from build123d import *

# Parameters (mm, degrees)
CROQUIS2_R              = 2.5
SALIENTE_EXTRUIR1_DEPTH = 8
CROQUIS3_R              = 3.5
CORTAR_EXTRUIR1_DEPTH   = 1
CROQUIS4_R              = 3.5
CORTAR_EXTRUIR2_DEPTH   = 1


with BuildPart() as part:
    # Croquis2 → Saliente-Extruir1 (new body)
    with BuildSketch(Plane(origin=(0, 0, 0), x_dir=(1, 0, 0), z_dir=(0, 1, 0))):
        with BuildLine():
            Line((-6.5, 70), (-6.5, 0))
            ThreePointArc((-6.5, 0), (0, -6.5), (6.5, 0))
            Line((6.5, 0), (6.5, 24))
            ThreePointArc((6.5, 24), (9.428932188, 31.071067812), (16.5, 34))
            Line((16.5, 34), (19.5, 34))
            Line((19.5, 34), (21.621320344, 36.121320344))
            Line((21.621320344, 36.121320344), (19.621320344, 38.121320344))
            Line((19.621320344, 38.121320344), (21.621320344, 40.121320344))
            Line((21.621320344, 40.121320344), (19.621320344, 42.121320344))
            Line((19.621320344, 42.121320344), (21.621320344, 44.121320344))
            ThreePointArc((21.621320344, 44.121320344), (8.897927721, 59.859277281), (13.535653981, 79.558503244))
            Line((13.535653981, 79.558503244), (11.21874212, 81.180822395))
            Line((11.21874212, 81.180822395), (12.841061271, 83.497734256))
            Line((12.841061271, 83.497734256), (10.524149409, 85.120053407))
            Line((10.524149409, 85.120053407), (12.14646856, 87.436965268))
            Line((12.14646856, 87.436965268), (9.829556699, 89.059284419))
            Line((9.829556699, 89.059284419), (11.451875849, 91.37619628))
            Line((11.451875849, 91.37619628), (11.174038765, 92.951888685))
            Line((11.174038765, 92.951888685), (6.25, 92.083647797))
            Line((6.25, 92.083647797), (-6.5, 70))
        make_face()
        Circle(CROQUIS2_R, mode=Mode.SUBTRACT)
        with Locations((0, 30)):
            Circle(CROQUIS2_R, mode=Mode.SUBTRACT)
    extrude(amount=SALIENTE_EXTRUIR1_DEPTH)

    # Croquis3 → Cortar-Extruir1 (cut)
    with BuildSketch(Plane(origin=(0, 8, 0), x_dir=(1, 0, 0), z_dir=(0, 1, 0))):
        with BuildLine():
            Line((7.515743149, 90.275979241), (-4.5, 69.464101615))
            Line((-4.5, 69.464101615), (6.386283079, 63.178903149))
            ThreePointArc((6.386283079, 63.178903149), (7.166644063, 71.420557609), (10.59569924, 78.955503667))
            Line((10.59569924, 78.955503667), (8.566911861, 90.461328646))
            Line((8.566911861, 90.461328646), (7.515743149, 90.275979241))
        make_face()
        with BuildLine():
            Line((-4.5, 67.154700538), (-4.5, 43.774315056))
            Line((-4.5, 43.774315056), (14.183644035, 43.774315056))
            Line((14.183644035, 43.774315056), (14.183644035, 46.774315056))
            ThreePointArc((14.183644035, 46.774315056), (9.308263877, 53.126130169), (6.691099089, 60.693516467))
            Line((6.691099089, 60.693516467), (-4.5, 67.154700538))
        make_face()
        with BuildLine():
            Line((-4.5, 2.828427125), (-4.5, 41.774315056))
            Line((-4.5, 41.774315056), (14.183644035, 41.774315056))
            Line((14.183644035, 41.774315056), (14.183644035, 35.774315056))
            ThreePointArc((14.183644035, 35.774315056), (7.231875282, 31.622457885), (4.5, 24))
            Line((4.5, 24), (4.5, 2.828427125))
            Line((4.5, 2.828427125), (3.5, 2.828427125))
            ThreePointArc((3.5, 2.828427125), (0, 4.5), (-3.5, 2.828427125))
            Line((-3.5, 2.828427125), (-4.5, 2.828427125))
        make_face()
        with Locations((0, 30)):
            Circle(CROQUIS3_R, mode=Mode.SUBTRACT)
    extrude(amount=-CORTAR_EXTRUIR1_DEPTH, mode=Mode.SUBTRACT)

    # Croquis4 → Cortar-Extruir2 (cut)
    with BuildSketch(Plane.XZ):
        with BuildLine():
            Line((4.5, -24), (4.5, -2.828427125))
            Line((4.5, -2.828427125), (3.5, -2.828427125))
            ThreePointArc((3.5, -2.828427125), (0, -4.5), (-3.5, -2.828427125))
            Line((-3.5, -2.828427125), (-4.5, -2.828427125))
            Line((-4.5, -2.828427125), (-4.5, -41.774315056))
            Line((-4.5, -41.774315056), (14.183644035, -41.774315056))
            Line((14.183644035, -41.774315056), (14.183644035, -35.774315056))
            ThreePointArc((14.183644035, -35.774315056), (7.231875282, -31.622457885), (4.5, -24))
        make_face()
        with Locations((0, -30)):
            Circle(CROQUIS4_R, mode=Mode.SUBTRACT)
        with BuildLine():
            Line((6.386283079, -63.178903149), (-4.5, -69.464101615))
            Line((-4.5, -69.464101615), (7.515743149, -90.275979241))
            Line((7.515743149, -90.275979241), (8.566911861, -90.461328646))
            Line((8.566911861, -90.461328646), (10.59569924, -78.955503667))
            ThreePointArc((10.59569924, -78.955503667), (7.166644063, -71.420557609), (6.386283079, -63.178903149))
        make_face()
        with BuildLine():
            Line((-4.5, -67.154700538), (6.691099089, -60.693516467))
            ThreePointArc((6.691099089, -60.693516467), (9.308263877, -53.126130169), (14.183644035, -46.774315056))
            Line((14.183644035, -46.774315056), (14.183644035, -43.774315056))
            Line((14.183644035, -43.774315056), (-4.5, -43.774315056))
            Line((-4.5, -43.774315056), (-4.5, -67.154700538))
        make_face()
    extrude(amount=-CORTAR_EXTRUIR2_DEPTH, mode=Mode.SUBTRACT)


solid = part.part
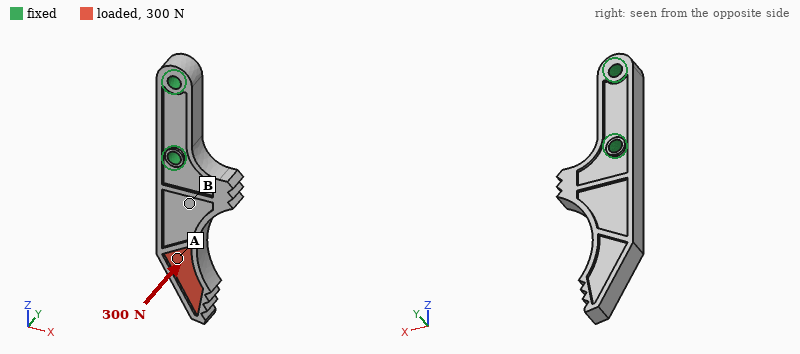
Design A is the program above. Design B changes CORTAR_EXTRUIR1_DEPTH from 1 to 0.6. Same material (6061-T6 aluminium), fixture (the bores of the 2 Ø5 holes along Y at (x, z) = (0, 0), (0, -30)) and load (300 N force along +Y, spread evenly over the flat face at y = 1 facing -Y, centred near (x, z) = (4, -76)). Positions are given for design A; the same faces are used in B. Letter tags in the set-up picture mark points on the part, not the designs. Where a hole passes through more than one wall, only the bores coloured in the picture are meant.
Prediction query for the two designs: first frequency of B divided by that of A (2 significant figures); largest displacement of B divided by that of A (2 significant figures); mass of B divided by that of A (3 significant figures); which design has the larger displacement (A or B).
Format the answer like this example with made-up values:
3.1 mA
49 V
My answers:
1.0
0.88
1.03
A
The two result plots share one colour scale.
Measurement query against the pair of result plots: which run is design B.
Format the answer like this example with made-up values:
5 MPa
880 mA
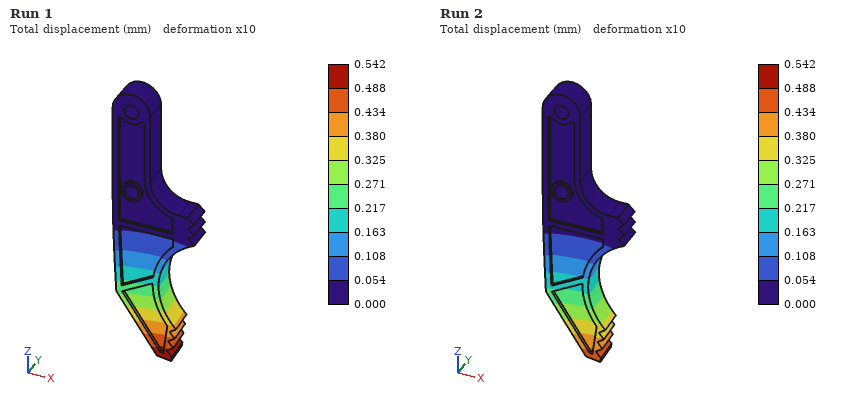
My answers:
Run 2
